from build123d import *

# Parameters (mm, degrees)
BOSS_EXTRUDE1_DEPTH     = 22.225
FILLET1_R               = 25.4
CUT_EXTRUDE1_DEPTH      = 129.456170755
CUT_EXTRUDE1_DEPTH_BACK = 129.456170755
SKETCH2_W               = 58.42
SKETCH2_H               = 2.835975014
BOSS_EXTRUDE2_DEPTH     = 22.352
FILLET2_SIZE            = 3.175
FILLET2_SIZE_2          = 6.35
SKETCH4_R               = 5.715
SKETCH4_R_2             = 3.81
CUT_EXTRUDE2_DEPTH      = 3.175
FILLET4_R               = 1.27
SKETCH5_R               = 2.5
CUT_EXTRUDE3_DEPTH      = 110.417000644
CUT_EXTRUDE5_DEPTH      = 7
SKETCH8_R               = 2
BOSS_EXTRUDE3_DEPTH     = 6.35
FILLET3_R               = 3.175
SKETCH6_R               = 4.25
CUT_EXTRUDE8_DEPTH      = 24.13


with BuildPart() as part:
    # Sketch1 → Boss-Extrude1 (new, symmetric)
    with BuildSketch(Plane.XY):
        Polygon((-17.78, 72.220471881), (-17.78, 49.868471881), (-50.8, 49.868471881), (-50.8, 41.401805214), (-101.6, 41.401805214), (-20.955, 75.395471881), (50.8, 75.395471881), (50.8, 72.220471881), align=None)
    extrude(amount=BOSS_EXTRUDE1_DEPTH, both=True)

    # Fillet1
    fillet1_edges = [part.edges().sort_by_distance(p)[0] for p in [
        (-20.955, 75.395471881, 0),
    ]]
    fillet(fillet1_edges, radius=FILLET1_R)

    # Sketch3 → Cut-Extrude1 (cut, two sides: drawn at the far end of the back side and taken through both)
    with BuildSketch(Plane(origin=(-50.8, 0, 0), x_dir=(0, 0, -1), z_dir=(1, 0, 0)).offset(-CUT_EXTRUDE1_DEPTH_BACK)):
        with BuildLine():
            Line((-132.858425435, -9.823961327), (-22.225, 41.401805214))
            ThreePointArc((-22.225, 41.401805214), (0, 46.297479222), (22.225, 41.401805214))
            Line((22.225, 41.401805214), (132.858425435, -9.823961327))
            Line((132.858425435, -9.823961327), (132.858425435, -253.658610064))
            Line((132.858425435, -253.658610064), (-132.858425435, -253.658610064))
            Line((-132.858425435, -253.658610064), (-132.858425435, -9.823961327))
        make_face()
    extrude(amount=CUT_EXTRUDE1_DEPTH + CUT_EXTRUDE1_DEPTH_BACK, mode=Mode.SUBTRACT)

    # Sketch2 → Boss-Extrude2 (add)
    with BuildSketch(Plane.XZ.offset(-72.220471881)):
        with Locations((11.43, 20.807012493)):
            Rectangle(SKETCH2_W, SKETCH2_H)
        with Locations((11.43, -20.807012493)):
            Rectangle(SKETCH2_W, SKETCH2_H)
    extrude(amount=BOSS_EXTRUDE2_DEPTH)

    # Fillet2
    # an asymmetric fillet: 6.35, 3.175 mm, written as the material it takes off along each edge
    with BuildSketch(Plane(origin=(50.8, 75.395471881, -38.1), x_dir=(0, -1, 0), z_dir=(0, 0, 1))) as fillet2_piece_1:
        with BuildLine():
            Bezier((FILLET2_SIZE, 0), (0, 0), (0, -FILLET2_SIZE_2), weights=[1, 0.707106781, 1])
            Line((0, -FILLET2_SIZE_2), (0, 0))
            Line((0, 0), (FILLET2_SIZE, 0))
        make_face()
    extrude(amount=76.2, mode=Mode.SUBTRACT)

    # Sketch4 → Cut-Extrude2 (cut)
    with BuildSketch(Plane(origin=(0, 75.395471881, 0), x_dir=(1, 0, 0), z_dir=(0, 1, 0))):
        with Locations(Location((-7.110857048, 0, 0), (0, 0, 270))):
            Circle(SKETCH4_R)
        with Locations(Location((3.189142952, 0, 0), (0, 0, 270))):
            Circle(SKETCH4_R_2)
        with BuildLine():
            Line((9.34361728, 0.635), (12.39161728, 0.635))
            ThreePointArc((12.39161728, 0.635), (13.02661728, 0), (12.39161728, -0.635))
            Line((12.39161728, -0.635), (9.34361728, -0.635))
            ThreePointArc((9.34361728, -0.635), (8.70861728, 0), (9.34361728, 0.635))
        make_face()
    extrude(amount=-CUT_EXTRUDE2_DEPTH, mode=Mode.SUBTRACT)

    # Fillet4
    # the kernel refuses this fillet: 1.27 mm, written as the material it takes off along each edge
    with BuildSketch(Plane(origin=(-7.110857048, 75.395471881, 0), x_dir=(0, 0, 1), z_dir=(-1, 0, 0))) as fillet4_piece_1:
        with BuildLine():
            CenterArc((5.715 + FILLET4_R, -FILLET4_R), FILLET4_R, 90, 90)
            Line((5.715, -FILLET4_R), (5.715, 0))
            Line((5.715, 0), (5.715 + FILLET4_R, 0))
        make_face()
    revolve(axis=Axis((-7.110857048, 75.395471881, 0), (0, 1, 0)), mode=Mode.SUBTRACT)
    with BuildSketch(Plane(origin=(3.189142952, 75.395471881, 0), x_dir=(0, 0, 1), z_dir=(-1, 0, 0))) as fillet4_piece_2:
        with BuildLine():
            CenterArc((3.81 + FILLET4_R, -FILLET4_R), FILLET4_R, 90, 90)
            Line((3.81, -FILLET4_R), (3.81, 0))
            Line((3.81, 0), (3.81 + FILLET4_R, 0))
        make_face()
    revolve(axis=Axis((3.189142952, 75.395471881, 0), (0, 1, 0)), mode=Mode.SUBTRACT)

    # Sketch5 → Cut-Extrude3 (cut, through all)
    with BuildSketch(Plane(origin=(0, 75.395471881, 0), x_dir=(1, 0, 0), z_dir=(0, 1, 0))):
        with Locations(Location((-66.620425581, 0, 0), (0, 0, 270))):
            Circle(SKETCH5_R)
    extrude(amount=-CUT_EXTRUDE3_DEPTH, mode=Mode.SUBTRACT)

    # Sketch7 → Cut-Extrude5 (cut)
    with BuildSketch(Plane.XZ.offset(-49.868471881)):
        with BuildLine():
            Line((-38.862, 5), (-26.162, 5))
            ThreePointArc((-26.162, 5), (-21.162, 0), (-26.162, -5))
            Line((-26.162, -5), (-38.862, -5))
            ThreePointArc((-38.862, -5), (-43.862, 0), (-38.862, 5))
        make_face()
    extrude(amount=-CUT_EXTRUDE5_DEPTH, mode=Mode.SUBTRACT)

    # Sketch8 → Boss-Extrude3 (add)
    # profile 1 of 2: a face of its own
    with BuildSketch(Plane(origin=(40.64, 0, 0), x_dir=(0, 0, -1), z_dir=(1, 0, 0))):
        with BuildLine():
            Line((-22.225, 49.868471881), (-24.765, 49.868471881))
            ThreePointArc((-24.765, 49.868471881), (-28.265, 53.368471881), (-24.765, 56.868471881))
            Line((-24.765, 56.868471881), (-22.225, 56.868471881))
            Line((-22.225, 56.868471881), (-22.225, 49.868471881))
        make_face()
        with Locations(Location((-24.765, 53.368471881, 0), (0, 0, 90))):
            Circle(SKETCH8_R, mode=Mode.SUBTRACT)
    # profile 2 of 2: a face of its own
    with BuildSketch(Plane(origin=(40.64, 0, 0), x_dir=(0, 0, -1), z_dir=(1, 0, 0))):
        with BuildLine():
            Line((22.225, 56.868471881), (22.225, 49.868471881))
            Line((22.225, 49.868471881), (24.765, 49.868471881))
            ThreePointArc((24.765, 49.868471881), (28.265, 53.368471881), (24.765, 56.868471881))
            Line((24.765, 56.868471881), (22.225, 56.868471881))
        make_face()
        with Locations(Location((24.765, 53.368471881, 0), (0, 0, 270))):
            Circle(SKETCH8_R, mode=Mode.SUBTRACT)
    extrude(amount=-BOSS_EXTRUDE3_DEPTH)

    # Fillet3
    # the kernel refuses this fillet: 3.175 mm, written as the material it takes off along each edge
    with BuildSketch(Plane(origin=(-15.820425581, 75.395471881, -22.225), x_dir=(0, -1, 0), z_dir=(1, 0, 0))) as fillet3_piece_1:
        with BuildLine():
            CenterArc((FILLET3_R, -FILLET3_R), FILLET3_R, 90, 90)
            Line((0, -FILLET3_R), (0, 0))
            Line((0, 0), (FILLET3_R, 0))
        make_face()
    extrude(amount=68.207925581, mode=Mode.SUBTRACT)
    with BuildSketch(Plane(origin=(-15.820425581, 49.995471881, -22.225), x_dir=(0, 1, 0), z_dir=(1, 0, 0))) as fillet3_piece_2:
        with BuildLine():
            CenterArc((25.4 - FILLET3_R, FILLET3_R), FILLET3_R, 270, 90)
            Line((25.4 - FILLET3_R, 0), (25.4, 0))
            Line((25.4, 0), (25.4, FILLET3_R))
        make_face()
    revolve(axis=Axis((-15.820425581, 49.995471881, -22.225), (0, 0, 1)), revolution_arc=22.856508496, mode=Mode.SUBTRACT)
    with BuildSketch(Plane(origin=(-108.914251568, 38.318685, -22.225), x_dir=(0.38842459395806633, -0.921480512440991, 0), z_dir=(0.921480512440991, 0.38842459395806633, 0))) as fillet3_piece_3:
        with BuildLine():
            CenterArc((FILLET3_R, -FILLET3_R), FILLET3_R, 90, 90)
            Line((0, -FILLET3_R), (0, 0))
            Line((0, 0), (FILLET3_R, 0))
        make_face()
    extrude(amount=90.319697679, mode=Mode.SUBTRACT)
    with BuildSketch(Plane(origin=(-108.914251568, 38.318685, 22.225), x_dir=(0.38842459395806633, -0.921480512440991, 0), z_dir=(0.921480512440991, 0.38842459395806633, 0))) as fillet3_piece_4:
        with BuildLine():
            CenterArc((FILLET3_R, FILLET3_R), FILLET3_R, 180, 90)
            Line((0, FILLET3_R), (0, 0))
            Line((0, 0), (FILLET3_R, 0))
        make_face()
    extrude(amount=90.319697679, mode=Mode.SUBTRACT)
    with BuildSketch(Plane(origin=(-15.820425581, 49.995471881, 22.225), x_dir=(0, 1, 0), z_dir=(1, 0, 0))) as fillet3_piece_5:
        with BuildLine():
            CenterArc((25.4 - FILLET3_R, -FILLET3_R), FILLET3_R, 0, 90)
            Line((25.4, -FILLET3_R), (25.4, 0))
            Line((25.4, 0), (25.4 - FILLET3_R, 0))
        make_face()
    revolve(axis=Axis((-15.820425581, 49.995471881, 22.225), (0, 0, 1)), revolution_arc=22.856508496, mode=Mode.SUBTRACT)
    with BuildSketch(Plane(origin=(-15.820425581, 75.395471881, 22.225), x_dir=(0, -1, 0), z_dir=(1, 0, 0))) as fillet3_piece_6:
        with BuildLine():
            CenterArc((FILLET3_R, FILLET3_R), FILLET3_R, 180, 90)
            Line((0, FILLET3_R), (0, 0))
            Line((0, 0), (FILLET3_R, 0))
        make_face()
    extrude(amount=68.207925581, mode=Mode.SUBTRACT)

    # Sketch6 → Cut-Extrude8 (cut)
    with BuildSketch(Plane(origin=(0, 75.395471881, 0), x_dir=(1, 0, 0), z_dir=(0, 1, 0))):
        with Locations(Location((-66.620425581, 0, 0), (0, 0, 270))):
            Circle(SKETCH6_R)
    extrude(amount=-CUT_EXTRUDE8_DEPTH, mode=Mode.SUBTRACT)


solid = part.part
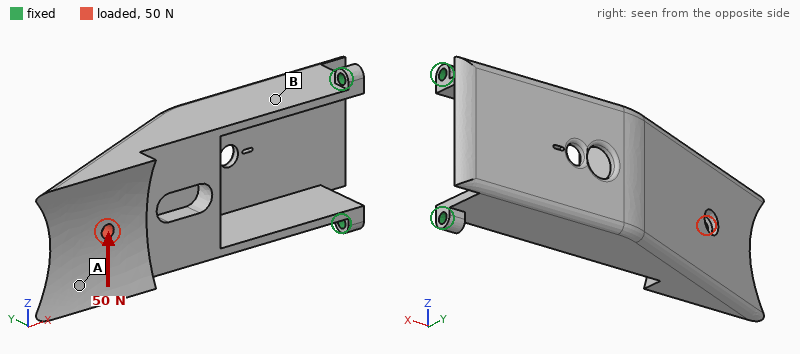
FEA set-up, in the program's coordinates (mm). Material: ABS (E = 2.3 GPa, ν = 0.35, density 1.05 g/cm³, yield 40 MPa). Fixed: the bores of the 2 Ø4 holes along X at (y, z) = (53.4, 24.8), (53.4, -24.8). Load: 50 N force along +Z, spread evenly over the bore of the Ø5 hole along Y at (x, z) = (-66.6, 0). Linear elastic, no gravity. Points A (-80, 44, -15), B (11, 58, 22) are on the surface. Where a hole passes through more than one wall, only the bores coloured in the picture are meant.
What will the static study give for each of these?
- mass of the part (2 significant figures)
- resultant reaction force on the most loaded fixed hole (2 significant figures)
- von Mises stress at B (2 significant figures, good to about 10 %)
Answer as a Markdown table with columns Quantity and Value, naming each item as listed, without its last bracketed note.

| Quantity | Value |
|---|---|
| mass of the part | 64 g |
| resultant reaction force on the most loaded fixed hole | 120 N |
| von Mises stress at B | 4.8 MPa |
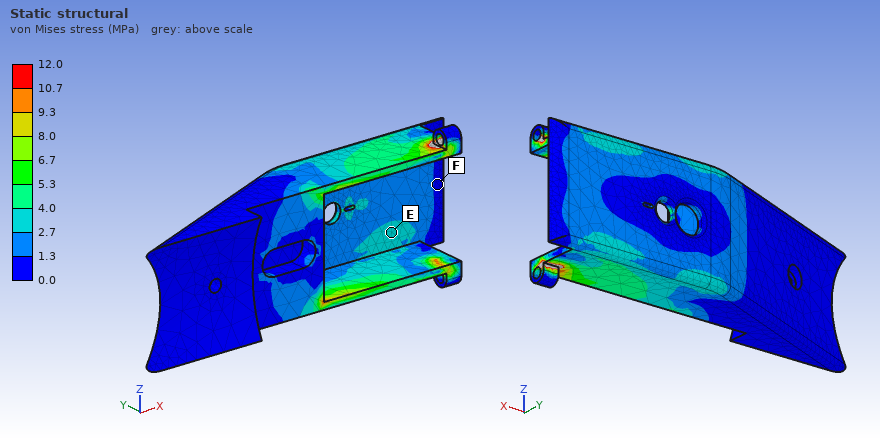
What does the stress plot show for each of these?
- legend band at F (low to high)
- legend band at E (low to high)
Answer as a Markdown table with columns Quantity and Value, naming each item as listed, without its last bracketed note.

| Quantity | Value |
|---|---|
| legend band at F | 0.0 to 1.3 MPa |
| legend band at E | 2.7 to 4.0 MPa |
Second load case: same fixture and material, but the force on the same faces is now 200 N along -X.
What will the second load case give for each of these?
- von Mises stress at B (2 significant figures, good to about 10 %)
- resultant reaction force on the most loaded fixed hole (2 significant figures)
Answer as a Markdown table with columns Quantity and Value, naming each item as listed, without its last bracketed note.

| Quantity | Value |
|---|---|
| von Mises stress at B | 3.0 MPa |
| resultant reaction force on the most loaded fixed hole | 100 N |
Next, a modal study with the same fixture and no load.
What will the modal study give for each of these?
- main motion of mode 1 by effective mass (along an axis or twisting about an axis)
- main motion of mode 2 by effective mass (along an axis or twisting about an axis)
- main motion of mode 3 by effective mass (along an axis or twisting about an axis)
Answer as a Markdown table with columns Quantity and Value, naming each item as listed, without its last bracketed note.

| Quantity | Value |
|---|---|
| main motion of mode 1 by effective mass | along Y |
| main motion of mode 2 by effective mass | along Z |
| main motion of mode 3 by effective mass | along Z |
